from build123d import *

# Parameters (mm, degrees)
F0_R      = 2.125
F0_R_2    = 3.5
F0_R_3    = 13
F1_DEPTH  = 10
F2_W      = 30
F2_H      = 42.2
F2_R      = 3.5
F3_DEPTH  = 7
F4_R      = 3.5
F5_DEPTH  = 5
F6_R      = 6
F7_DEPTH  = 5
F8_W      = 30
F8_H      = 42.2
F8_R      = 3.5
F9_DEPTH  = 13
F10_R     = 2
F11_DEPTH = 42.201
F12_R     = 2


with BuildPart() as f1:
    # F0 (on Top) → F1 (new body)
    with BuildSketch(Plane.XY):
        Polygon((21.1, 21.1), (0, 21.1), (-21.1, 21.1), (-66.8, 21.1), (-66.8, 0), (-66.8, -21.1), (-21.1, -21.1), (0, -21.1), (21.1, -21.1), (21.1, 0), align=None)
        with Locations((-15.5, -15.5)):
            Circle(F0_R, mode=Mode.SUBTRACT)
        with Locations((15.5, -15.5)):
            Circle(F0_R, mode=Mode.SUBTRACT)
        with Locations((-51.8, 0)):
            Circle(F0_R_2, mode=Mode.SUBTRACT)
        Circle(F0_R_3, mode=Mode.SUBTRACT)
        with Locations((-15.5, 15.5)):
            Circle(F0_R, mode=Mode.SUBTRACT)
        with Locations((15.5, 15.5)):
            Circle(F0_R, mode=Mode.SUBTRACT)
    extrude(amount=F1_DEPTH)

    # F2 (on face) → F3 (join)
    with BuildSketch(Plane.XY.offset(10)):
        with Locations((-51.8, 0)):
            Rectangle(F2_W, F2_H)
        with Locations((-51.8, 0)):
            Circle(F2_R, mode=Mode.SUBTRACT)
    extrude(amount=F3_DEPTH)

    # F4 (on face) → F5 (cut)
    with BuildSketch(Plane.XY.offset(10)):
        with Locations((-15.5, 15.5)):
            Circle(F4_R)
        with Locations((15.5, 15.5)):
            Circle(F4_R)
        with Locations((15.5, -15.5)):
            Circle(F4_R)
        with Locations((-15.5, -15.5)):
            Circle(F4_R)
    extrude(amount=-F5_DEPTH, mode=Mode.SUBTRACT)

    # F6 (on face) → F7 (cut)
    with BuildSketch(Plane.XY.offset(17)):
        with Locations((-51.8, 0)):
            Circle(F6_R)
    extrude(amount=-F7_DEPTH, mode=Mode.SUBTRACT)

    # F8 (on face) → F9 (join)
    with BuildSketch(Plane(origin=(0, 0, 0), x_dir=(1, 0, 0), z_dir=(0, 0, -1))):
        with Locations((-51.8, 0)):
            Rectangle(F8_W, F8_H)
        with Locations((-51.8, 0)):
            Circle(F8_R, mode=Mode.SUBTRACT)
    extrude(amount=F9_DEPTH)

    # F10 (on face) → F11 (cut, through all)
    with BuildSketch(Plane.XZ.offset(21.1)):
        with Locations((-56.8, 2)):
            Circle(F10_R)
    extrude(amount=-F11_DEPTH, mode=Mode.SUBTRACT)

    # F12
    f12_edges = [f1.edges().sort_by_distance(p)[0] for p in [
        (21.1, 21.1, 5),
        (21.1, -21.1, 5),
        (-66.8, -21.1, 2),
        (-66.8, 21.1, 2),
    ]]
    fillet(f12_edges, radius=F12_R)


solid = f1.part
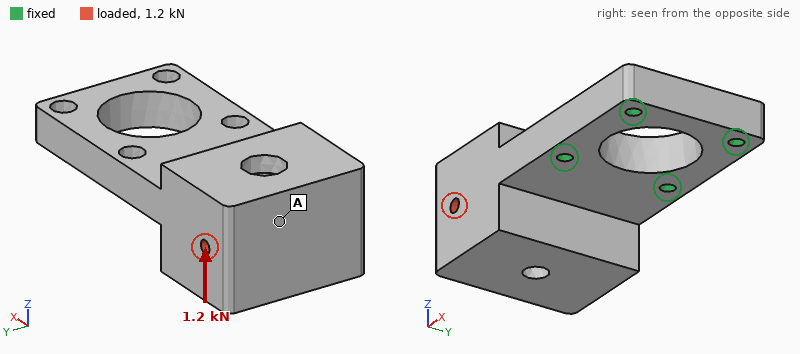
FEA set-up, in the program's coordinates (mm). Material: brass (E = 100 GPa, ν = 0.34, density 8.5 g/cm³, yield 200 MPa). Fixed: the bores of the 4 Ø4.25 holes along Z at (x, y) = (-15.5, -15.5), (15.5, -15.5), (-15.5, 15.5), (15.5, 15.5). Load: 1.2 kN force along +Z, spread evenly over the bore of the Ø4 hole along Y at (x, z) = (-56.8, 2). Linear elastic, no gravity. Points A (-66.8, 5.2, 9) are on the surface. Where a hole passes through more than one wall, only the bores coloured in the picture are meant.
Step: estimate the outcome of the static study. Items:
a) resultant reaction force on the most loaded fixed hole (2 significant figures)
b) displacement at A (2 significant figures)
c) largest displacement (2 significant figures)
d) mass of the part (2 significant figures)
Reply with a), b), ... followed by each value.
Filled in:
a) 1.3 kN
b) 0.19 mm
c) 0.20 mm
d) 460 g
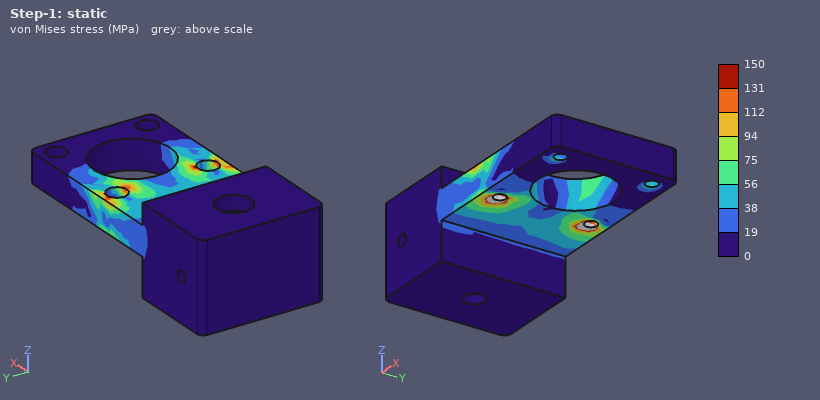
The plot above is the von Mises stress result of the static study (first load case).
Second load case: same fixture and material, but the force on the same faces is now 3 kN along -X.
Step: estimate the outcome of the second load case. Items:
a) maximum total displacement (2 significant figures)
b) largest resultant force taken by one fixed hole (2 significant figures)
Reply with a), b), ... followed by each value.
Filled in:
a) 30 µm
b) 1.5 kN
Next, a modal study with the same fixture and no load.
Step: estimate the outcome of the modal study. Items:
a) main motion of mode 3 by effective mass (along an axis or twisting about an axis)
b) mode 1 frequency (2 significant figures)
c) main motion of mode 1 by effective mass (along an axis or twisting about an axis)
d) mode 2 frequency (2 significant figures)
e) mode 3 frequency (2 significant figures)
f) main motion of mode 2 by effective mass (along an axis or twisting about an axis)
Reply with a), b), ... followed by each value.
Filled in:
a) along Y
b) 890 Hz
c) along Z
d) 2900 Hz
e) 4000 Hz
f) along Y
